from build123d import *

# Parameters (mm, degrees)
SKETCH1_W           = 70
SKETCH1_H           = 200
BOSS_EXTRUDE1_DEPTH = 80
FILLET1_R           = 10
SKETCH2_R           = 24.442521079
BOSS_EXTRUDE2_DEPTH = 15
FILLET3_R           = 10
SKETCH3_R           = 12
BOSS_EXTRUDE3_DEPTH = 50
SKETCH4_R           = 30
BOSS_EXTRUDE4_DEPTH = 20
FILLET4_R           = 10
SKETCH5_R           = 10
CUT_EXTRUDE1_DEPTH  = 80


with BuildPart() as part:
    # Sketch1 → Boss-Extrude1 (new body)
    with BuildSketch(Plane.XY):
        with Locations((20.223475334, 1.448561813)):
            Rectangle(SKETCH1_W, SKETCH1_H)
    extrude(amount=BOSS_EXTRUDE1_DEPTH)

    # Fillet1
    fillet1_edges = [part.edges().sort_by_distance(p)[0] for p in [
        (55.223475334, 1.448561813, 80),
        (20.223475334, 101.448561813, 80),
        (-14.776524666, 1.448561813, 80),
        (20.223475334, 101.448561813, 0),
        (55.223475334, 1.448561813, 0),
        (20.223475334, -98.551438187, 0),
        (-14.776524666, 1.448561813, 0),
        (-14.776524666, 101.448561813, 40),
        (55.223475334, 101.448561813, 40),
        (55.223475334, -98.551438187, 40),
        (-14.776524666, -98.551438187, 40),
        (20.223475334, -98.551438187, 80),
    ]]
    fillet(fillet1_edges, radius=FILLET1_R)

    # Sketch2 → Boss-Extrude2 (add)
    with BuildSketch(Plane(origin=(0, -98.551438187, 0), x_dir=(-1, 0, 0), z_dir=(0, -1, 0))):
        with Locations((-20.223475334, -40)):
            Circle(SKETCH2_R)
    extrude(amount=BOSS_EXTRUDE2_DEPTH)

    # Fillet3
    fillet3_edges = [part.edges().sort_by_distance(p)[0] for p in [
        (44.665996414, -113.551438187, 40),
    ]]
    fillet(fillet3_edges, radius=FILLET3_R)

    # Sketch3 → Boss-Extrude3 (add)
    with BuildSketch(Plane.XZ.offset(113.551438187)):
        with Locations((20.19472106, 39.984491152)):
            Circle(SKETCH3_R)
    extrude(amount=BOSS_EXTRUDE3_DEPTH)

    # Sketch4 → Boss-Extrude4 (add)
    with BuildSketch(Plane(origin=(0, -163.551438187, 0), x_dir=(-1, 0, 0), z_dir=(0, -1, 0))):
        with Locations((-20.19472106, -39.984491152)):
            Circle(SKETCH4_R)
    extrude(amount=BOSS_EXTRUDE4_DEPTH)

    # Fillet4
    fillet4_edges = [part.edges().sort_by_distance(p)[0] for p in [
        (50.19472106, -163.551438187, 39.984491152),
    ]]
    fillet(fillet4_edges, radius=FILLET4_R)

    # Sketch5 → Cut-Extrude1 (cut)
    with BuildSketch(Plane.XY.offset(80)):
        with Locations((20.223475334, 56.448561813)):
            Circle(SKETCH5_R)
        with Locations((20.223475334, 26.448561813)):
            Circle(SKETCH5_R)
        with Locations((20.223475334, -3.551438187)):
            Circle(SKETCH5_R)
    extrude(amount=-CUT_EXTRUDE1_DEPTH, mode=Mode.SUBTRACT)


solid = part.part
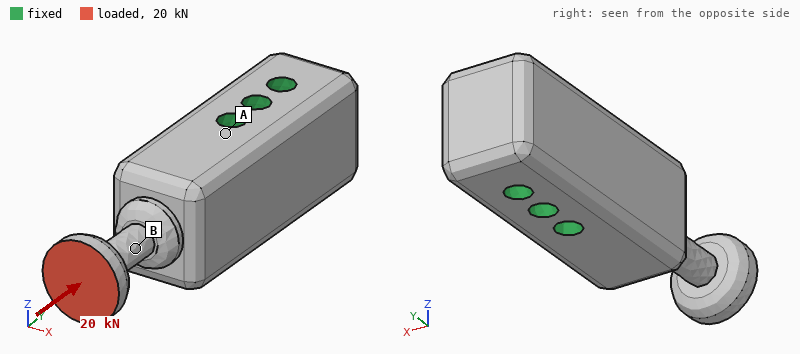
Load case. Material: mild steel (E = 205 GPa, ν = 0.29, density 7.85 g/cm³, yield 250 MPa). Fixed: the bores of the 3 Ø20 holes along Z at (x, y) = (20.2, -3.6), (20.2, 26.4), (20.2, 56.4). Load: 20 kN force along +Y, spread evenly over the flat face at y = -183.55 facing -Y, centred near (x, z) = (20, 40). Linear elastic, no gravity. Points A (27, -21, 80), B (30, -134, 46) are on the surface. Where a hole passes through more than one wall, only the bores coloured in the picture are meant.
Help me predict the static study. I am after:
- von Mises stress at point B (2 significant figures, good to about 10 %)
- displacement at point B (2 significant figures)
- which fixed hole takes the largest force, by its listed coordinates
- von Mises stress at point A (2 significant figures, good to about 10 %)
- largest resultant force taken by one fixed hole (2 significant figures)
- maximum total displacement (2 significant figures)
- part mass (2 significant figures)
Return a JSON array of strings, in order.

["43 MPa", "8.6 µm", "(20.2, -3.6)", "5.4 MPa", "16 kN", "19 µm", "8.8 kg"]
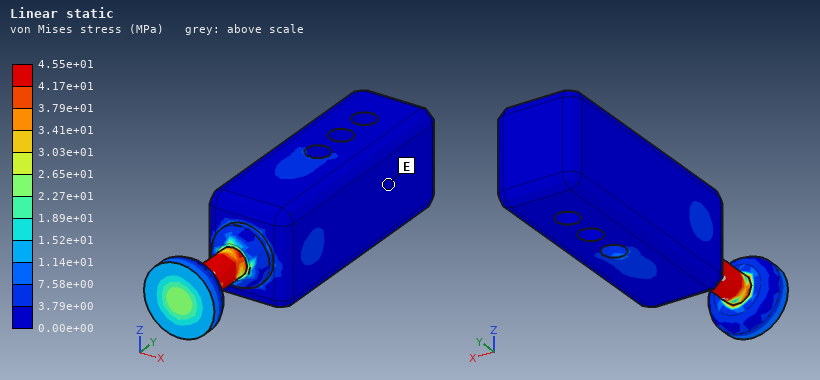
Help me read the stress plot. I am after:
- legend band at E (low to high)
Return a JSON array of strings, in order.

["0.00e+00 to 3.79e+00 MPa"]
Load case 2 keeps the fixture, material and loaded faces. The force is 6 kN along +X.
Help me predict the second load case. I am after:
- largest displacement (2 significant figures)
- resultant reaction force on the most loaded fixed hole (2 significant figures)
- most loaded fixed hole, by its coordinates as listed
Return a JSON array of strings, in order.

["0.34 mm", "18 kN", "(20.2, -3.6)"]
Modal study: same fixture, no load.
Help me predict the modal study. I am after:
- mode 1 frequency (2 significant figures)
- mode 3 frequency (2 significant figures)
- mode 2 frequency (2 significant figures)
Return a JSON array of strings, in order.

["1200 Hz", "2500 Hz", "1200 Hz"]
